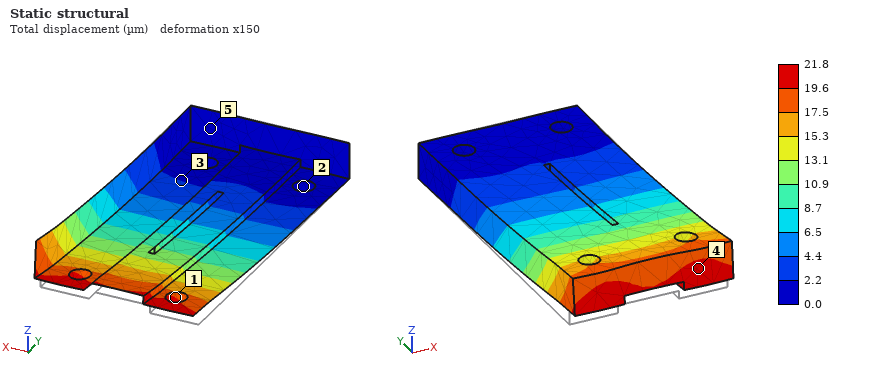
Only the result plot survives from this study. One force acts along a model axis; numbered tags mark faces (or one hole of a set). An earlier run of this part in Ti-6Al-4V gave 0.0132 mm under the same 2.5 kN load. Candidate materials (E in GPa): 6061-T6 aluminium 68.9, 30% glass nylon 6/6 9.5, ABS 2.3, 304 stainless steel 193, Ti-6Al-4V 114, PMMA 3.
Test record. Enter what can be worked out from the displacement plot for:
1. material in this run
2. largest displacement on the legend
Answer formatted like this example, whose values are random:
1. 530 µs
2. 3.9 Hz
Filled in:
1. 6061-T6 aluminium
2. 21.8 µm
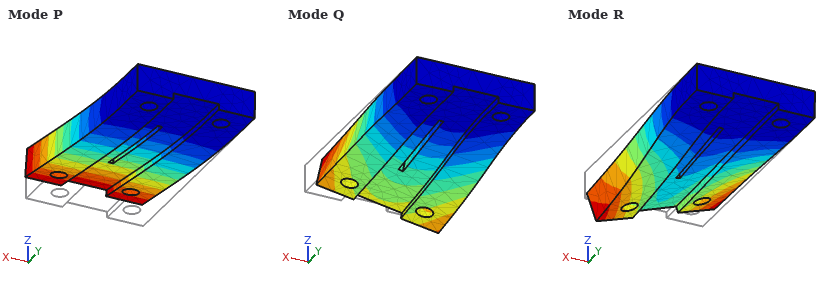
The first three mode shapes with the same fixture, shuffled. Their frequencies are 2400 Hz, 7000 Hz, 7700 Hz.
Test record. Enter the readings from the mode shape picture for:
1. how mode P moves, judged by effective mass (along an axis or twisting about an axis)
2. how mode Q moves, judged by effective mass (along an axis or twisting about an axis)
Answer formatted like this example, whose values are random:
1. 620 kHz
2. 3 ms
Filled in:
1. along Z
2. along X
